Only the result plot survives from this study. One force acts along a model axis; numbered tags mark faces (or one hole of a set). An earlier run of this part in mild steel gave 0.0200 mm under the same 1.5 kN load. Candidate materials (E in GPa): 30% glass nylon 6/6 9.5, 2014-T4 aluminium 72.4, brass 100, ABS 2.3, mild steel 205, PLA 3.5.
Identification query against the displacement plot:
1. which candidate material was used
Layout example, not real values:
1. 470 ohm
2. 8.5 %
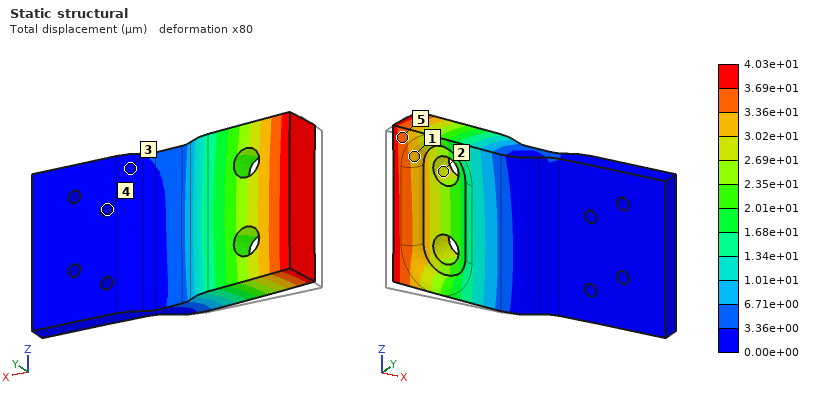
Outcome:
1. brass
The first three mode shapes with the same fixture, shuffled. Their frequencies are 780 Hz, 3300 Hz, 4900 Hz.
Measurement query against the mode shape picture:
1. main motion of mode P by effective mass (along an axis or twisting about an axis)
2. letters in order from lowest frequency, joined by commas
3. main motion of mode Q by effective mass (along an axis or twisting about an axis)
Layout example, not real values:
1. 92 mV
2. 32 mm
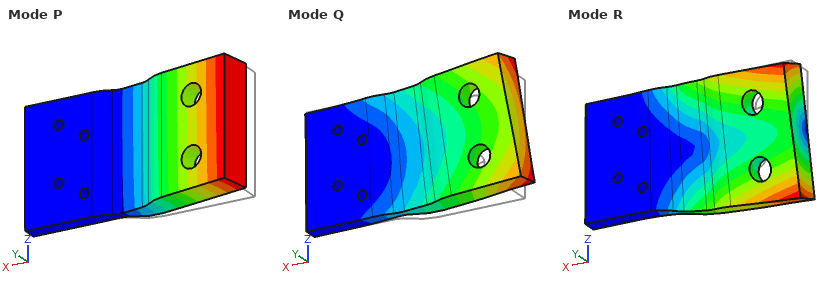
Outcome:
1. along Y
2. P, R, Q
3. along Z
